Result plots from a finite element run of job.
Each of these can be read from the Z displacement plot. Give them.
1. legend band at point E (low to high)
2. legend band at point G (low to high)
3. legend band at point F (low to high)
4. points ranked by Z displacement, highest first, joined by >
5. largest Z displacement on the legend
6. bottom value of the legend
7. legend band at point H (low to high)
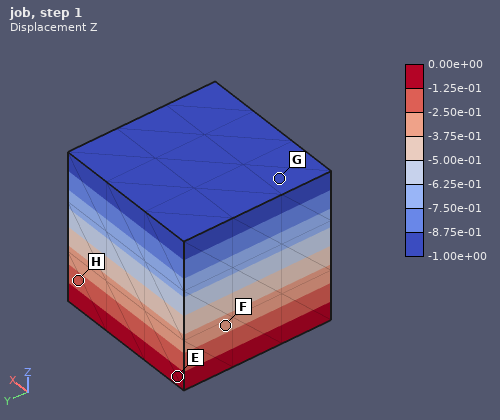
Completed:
-1.25e-01 to 0.00e+00
-1.00e+00 to -8.75e-01
-3.75e-01 to -2.50e-01
E > H > F > G
0.00e+00
-1.00e+00
-2.50e-01 to -1.25e-01
